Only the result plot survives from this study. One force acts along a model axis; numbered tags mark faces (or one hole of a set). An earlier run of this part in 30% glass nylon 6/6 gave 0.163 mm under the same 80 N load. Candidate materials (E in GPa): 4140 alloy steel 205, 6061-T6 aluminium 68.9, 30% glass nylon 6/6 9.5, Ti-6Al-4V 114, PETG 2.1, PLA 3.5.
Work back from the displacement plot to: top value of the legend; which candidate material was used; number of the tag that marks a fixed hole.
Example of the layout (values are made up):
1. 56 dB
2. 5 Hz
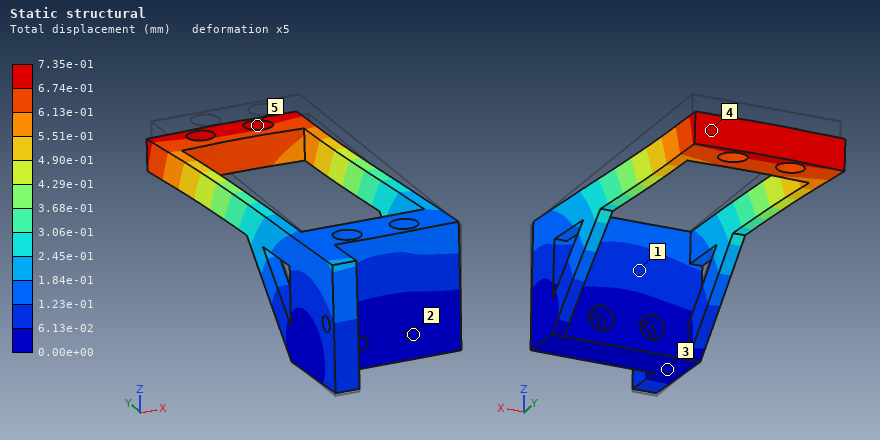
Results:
1. 7.35e-01 mm
2. PETG
3. 2
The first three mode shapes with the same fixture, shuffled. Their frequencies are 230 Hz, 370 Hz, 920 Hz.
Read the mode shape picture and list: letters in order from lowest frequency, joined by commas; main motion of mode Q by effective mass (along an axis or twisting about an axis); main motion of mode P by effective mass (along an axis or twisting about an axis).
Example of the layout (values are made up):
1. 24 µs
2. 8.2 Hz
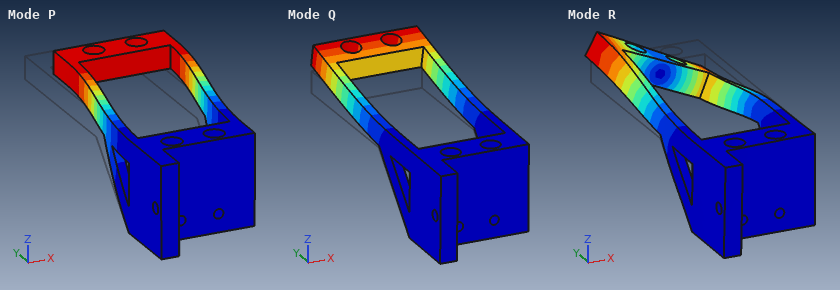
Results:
1. P, Q, R
2. along Z
3. along X
